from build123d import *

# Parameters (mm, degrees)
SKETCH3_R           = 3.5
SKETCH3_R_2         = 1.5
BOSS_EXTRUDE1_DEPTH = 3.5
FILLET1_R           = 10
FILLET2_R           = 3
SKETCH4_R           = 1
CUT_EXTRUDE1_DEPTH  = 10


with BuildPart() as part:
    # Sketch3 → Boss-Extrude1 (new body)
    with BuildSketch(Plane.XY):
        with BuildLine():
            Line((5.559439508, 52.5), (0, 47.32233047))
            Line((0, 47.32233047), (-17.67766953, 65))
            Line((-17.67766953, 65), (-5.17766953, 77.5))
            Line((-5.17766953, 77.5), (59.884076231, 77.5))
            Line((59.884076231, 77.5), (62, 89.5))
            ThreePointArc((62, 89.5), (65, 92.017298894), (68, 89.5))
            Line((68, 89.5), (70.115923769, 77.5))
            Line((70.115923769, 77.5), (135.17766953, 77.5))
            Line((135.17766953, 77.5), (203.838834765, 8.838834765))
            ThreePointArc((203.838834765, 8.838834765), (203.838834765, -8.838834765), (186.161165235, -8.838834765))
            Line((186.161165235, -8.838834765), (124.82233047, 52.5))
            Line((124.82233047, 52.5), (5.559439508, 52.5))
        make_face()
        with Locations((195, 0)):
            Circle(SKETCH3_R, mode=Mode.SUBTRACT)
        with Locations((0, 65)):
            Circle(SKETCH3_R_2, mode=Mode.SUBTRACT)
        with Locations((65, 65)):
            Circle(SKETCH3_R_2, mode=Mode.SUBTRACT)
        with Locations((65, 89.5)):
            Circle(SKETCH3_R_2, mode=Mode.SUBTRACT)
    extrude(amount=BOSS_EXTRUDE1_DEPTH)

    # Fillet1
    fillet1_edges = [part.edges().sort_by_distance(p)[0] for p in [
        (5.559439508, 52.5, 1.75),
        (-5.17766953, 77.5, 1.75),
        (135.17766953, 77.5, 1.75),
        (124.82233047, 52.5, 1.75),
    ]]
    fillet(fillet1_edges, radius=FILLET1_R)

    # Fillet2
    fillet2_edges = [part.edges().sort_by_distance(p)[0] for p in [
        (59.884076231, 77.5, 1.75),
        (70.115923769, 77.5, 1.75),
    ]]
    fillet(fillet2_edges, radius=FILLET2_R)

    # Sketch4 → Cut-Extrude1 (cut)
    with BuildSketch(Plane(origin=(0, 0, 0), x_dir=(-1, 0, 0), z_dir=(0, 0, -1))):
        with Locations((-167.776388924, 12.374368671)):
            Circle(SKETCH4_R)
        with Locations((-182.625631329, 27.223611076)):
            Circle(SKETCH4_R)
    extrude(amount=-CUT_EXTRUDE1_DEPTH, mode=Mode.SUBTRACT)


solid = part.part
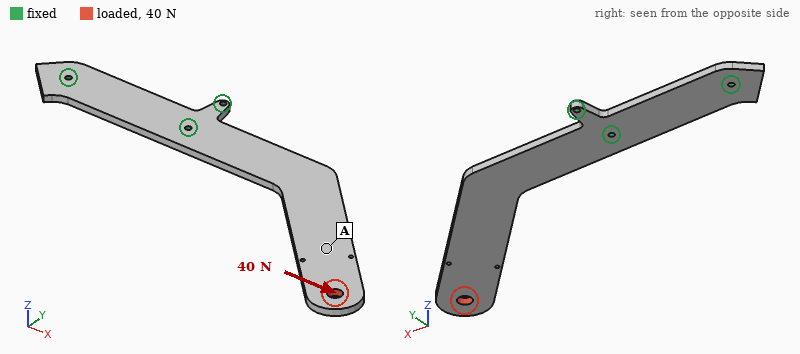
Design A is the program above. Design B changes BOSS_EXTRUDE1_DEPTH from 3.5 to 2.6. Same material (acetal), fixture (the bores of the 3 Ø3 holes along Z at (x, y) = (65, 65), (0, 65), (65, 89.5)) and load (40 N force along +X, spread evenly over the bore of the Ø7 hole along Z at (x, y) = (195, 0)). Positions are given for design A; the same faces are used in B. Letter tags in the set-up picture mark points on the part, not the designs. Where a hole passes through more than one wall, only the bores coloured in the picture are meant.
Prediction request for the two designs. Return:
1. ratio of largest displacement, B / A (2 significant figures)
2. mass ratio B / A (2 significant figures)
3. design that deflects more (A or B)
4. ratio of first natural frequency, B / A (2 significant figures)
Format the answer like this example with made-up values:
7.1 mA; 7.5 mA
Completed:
1.3; 0.74; B; 0.75
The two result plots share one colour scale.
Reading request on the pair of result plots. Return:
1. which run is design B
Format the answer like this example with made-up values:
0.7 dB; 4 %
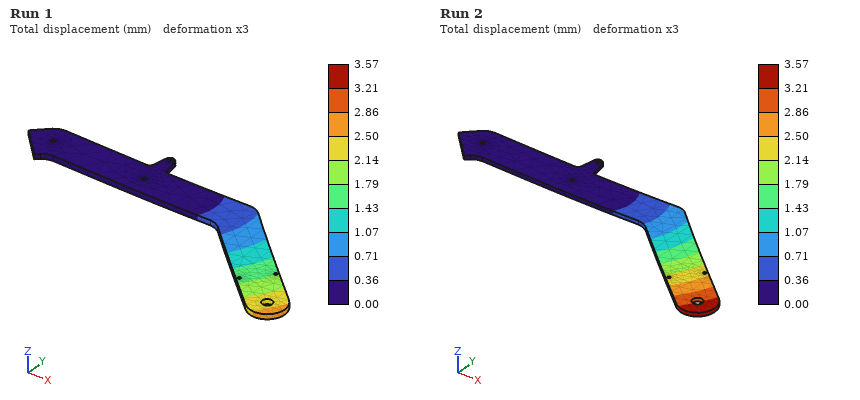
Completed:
Run 2
